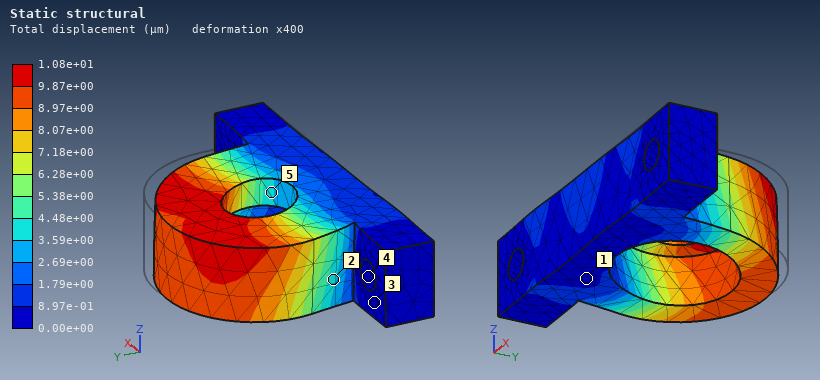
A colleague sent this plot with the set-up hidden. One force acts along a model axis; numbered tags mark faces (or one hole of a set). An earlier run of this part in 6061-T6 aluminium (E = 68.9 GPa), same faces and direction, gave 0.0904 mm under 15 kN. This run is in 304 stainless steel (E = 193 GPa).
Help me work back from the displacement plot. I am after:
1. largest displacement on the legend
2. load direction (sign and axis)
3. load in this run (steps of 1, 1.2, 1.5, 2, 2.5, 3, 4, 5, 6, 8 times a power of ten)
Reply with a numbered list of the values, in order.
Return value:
1. 1.08e+01 µm
2. -X
3. 5 kN
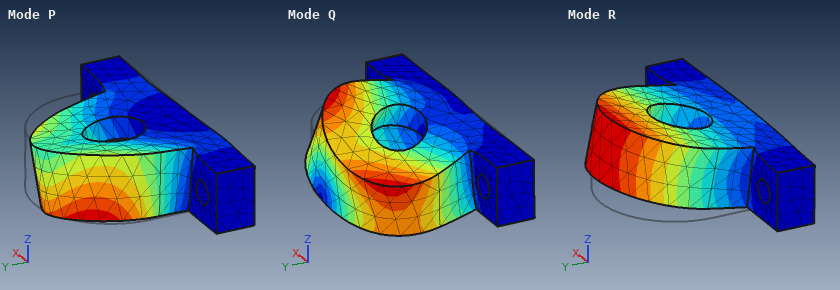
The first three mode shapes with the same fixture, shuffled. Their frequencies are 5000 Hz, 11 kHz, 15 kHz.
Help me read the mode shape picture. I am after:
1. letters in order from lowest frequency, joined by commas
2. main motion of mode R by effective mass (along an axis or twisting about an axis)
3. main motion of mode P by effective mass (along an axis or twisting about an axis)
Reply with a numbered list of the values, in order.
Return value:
1. R, P, Q
2. along Z
3. along X
